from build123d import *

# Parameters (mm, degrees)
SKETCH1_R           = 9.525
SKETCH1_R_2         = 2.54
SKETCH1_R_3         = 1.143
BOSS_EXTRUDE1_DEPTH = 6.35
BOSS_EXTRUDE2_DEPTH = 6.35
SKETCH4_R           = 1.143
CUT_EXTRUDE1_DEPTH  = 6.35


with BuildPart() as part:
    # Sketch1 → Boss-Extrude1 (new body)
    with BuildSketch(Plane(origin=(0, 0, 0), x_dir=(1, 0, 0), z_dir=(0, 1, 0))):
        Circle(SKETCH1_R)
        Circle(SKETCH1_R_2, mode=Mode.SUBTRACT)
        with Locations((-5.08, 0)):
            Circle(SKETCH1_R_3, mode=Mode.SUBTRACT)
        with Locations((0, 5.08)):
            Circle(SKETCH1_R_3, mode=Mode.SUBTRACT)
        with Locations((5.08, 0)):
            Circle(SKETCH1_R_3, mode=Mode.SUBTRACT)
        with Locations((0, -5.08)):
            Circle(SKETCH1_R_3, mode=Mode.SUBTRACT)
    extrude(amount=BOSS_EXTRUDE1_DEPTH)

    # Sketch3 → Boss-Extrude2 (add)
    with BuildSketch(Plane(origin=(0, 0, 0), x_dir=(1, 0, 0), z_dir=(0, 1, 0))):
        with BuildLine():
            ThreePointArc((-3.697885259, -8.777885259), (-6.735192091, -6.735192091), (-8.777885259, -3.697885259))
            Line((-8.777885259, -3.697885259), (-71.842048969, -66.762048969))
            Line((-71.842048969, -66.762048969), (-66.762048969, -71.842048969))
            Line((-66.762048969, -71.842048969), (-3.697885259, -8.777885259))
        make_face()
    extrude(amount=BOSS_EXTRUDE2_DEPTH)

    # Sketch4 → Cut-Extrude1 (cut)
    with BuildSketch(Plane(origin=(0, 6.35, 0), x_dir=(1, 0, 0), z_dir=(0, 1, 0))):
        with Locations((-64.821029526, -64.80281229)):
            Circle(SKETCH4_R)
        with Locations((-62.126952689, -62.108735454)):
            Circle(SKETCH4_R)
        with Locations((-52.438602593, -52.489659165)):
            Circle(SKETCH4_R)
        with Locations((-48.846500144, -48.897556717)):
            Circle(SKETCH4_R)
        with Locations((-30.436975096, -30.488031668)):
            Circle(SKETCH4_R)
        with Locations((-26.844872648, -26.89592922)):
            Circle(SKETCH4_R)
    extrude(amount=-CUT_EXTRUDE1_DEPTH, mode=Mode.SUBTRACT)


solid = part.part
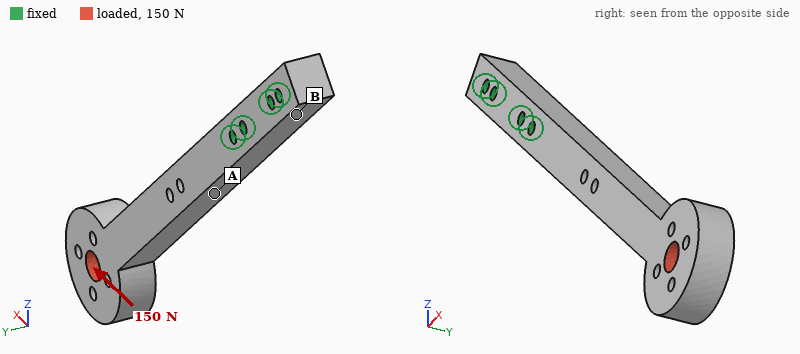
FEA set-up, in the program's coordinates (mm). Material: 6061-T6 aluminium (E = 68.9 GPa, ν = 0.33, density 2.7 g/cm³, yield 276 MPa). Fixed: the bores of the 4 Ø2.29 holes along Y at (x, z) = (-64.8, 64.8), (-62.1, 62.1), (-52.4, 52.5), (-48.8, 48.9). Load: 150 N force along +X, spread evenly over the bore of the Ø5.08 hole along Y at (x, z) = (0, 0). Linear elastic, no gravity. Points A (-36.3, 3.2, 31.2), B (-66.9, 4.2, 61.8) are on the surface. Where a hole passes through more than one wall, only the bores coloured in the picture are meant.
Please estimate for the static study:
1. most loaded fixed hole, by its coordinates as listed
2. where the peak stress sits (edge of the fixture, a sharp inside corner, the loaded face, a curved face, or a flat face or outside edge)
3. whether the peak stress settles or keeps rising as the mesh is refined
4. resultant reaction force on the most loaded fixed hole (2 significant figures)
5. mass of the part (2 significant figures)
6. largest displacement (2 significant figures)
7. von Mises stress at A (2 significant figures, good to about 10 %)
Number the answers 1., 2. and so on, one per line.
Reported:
1. (-48.8, 48.9)
2. edge of the fixture
3. keeps rising
4. 710 N
5. 15 g
6. 1.1 mm
7. 96 MPa
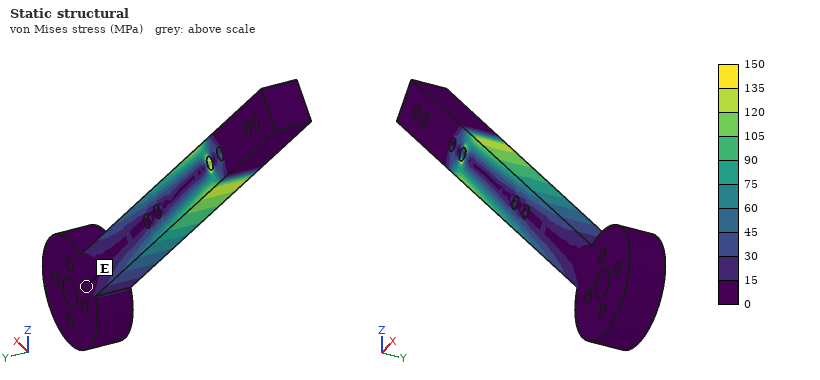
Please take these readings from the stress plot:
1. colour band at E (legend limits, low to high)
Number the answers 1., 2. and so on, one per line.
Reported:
1. 0 to 15 MPa
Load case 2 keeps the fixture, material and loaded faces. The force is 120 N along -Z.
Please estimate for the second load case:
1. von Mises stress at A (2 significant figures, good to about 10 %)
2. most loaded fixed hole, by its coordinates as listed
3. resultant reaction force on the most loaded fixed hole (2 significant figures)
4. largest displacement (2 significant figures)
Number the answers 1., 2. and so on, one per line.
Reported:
1. 73 MPa
2. (-48.8, 48.9)
3. 570 N
4. 0.90 mm
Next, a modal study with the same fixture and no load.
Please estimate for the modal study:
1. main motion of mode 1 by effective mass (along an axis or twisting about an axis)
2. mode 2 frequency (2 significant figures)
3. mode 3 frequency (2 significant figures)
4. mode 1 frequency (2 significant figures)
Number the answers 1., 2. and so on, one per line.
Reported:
1. along Y
2. 720 Hz
3. 4600 Hz
4. 650 Hz
